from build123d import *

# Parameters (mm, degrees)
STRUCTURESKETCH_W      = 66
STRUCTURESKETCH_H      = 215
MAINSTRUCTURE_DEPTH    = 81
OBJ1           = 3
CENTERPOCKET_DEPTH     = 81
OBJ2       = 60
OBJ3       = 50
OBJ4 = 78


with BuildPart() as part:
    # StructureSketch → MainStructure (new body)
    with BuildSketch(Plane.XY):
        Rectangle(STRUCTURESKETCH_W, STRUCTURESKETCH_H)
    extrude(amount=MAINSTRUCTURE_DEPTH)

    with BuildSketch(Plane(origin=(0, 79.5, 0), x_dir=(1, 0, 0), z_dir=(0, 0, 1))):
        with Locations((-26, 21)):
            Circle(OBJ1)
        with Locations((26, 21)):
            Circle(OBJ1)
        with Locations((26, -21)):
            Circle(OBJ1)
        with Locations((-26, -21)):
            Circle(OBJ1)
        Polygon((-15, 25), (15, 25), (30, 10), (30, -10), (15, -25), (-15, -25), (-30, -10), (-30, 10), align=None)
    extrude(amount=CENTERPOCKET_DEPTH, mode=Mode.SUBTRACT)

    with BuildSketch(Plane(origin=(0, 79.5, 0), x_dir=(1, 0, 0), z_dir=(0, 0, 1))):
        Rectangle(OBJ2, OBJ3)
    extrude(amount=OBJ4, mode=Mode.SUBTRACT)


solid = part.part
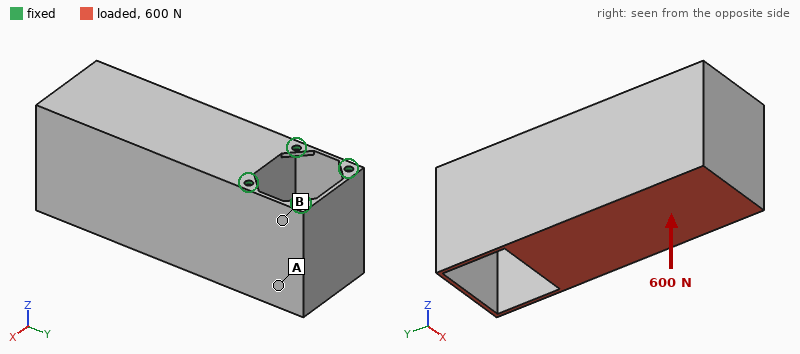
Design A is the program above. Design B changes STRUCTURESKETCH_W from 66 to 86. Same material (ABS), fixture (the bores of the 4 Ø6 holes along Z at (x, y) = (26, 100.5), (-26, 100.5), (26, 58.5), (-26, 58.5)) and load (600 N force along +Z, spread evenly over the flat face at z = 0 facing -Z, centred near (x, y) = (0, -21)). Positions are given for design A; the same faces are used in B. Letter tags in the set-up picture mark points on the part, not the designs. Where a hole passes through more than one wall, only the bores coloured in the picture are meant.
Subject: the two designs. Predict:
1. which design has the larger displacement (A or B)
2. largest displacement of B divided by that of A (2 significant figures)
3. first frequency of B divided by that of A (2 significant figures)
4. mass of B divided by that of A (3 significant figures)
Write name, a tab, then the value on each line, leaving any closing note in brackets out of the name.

which design has the larger displacement	A
largest displacement of B divided by that of A	0.59
first frequency of B divided by that of A	1.1
mass of B divided by that of A	1.38
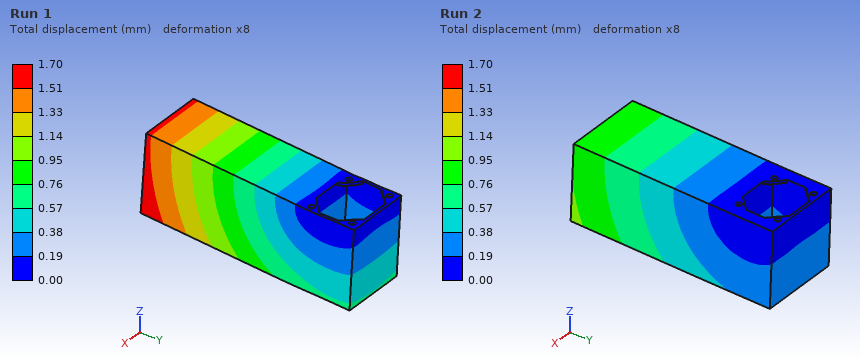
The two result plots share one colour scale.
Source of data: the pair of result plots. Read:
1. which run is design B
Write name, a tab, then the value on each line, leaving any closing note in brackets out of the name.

which run is design B	Run 2
